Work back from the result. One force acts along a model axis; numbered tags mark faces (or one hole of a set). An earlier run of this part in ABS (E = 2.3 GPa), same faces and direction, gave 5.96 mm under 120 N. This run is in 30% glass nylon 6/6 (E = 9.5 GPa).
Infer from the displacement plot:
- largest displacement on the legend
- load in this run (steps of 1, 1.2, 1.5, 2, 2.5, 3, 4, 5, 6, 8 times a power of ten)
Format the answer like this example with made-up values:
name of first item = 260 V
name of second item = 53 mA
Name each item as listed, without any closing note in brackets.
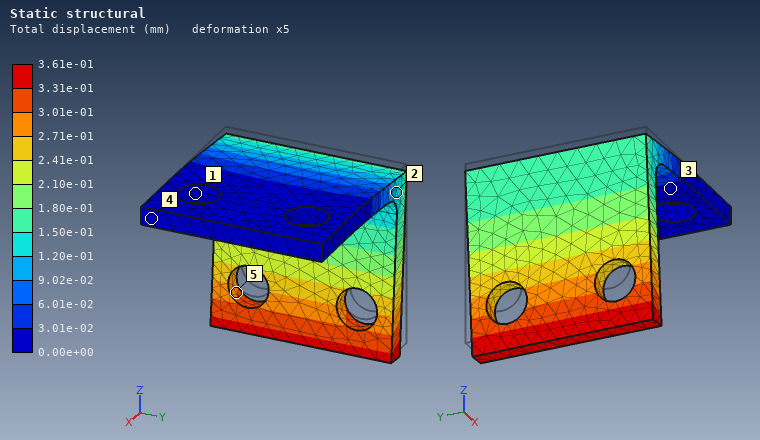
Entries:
largest displacement on the legend = 3.61e-01 mm
load in this run = 30 N
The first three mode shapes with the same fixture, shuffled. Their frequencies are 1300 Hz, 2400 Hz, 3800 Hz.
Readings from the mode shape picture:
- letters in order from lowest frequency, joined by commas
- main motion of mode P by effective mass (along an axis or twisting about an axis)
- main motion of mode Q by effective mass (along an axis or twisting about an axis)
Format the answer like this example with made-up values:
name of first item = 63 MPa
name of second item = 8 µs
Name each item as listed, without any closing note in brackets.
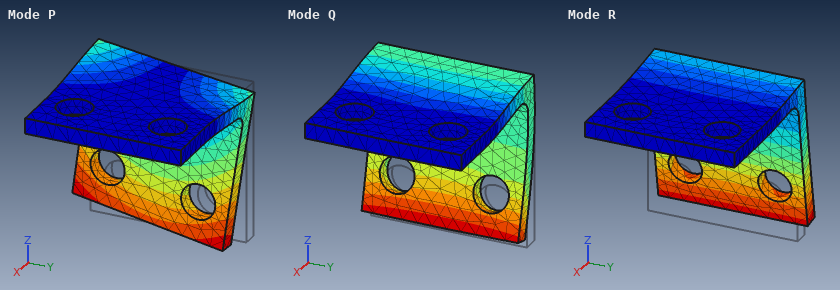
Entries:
letters in order from lowest frequency, joined by commas = R, P, Q
main motion of mode P by effective mass = along Y
main motion of mode Q by effective mass = along Z
